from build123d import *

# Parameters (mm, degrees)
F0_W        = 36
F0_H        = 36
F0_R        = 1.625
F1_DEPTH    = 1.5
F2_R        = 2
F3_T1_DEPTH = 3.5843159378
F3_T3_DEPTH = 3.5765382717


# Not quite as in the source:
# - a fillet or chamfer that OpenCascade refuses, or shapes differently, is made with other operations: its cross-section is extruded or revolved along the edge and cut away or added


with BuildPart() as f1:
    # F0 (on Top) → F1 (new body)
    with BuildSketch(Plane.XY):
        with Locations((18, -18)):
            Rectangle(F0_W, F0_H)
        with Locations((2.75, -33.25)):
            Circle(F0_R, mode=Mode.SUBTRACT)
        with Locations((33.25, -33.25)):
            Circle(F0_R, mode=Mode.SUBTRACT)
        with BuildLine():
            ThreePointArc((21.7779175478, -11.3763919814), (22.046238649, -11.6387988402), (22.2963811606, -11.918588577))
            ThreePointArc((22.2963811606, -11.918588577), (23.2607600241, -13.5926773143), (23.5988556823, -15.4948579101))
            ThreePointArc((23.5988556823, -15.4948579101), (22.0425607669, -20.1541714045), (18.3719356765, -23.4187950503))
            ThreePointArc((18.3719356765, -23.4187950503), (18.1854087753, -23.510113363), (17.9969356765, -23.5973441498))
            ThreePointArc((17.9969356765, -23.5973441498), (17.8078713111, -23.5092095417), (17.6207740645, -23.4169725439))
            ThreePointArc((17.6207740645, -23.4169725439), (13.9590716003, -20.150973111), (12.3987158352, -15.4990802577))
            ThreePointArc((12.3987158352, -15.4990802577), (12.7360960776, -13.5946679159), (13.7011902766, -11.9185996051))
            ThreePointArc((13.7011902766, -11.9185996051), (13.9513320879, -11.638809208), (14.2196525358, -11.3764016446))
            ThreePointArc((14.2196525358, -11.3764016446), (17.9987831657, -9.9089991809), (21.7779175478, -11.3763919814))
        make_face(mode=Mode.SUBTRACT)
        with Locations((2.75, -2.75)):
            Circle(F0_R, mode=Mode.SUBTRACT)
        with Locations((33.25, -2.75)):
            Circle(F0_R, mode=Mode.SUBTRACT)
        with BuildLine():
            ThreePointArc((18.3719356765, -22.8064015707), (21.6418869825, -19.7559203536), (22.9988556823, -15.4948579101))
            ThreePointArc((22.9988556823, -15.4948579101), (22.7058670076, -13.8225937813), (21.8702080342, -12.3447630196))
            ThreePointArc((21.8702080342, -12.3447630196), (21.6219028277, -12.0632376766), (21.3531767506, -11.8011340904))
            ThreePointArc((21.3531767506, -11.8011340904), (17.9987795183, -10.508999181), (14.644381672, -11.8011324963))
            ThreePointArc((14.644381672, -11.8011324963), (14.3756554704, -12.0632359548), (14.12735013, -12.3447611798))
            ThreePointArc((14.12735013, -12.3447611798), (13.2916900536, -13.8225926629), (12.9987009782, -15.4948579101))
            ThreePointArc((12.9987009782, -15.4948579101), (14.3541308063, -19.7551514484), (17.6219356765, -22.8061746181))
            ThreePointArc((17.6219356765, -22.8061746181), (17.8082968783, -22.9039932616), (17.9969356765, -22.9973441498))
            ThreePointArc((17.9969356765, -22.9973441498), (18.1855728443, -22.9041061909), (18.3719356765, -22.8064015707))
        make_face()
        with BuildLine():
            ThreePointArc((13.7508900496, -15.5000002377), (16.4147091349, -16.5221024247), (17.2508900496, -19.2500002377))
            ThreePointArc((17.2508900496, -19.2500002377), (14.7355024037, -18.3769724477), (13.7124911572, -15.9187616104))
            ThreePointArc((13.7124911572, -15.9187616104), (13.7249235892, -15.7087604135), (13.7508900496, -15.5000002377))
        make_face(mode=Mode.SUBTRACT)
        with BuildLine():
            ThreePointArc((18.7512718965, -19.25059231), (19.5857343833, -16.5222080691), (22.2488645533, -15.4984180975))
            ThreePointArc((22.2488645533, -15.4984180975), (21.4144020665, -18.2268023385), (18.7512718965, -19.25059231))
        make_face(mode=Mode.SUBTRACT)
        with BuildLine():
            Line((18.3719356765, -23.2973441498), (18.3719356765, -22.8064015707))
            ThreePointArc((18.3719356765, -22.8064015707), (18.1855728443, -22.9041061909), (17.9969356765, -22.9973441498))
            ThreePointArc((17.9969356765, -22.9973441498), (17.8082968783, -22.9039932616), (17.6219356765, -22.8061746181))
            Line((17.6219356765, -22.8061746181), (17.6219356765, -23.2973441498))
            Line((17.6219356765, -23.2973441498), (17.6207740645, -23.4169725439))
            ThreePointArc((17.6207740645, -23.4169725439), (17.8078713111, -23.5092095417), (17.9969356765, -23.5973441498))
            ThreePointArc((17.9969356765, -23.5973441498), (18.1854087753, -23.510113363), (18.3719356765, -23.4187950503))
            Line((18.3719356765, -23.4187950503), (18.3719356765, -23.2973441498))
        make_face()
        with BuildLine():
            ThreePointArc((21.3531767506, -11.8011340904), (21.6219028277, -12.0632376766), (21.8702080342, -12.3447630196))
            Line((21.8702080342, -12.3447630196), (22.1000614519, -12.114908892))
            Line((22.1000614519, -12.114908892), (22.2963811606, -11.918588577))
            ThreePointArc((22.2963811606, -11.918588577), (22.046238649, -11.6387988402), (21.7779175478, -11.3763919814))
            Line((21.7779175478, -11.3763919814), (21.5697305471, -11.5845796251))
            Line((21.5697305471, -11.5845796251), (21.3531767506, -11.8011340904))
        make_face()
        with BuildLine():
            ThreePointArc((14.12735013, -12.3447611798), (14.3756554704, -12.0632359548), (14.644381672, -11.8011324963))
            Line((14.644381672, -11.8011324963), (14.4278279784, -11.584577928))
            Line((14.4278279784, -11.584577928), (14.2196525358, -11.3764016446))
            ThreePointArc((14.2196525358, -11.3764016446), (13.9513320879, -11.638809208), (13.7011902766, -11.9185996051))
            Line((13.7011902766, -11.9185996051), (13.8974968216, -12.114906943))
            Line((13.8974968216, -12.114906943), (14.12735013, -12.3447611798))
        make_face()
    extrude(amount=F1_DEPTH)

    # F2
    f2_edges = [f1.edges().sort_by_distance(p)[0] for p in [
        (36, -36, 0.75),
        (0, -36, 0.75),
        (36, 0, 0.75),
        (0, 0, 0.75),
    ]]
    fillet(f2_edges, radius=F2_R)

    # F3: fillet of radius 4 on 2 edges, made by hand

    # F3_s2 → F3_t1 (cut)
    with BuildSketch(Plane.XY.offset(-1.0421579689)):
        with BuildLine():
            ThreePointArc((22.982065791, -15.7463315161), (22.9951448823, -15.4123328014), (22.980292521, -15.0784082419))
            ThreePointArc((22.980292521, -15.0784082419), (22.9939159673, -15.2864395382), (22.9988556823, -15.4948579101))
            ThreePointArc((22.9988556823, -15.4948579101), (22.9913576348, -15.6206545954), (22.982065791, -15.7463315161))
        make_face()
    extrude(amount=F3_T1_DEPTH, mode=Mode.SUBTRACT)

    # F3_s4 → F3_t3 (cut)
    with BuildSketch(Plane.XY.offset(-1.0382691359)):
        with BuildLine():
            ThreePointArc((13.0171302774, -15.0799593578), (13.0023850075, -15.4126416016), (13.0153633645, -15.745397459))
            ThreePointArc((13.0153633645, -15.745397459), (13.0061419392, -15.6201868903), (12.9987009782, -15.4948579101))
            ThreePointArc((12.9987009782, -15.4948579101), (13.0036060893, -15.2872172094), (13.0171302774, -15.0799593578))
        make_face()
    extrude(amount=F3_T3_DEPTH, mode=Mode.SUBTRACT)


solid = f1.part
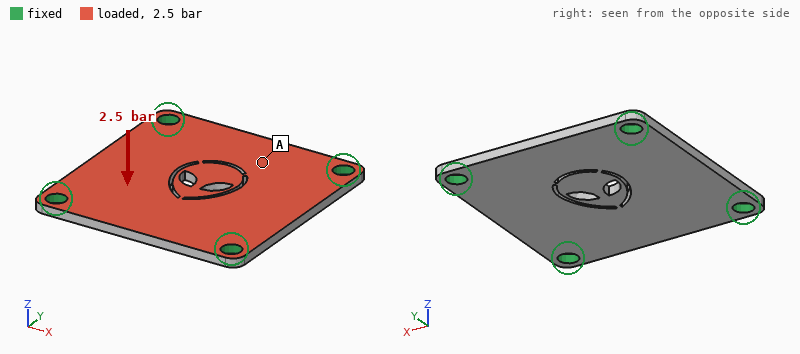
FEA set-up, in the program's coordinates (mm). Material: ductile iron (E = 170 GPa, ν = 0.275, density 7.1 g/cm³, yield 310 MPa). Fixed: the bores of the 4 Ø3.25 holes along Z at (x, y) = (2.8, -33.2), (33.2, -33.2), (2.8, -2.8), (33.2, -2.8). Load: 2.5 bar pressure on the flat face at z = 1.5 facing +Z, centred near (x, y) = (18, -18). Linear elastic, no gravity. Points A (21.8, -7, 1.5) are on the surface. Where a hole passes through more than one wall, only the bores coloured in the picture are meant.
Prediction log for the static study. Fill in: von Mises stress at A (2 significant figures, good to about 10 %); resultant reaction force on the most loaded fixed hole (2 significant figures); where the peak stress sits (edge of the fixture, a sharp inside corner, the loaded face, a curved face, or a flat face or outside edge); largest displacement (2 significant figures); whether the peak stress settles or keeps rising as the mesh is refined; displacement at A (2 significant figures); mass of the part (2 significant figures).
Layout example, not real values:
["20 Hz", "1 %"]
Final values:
["27 MPa", "76 N", "edge of the fixture", "31 µm", "keeps rising", "18 µm", "13 g"]
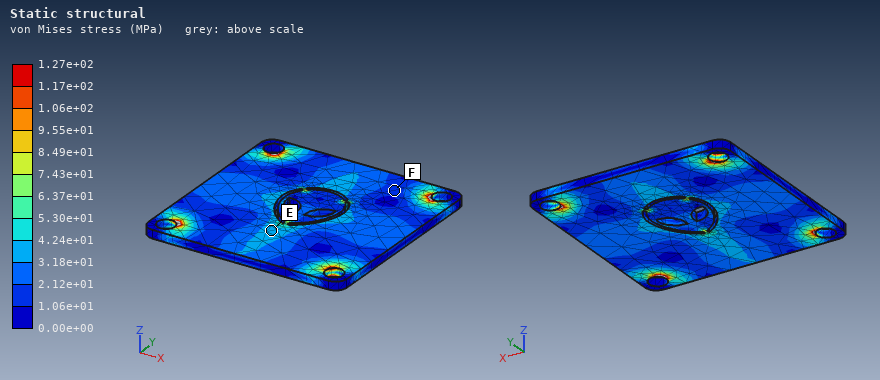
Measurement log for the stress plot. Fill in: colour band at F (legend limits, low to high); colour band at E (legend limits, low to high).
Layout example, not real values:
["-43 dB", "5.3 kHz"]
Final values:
["1.06e+01 to 2.12e+01 MPa", "3.18e+01 to 4.24e+01 MPa"]
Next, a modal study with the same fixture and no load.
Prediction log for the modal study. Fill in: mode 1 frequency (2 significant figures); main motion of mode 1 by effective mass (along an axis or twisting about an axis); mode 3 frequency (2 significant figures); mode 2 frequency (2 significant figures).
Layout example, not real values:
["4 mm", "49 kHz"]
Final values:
["5600 Hz", "along Z", "9700 Hz", "9700 Hz"]
